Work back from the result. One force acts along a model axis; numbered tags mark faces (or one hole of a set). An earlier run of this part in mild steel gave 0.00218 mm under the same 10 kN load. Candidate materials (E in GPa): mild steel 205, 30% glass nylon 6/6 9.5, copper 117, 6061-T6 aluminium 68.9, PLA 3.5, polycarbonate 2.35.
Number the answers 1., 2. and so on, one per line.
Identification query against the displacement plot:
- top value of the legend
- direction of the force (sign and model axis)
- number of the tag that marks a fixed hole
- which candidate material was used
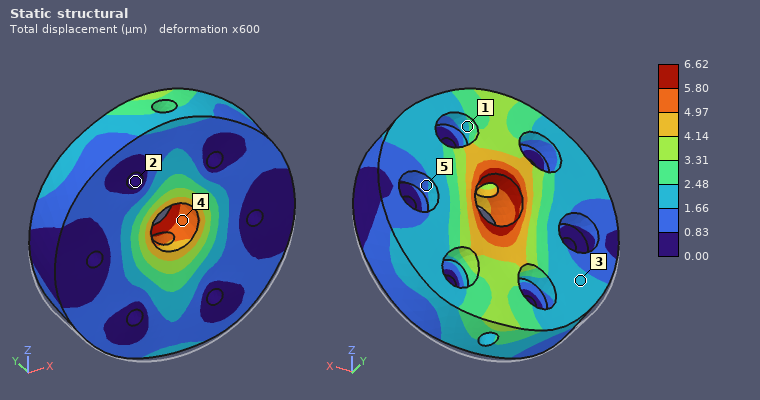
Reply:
1. 6.62 µm
2. +Z
3. 2
4. 6061-T6 aluminium
